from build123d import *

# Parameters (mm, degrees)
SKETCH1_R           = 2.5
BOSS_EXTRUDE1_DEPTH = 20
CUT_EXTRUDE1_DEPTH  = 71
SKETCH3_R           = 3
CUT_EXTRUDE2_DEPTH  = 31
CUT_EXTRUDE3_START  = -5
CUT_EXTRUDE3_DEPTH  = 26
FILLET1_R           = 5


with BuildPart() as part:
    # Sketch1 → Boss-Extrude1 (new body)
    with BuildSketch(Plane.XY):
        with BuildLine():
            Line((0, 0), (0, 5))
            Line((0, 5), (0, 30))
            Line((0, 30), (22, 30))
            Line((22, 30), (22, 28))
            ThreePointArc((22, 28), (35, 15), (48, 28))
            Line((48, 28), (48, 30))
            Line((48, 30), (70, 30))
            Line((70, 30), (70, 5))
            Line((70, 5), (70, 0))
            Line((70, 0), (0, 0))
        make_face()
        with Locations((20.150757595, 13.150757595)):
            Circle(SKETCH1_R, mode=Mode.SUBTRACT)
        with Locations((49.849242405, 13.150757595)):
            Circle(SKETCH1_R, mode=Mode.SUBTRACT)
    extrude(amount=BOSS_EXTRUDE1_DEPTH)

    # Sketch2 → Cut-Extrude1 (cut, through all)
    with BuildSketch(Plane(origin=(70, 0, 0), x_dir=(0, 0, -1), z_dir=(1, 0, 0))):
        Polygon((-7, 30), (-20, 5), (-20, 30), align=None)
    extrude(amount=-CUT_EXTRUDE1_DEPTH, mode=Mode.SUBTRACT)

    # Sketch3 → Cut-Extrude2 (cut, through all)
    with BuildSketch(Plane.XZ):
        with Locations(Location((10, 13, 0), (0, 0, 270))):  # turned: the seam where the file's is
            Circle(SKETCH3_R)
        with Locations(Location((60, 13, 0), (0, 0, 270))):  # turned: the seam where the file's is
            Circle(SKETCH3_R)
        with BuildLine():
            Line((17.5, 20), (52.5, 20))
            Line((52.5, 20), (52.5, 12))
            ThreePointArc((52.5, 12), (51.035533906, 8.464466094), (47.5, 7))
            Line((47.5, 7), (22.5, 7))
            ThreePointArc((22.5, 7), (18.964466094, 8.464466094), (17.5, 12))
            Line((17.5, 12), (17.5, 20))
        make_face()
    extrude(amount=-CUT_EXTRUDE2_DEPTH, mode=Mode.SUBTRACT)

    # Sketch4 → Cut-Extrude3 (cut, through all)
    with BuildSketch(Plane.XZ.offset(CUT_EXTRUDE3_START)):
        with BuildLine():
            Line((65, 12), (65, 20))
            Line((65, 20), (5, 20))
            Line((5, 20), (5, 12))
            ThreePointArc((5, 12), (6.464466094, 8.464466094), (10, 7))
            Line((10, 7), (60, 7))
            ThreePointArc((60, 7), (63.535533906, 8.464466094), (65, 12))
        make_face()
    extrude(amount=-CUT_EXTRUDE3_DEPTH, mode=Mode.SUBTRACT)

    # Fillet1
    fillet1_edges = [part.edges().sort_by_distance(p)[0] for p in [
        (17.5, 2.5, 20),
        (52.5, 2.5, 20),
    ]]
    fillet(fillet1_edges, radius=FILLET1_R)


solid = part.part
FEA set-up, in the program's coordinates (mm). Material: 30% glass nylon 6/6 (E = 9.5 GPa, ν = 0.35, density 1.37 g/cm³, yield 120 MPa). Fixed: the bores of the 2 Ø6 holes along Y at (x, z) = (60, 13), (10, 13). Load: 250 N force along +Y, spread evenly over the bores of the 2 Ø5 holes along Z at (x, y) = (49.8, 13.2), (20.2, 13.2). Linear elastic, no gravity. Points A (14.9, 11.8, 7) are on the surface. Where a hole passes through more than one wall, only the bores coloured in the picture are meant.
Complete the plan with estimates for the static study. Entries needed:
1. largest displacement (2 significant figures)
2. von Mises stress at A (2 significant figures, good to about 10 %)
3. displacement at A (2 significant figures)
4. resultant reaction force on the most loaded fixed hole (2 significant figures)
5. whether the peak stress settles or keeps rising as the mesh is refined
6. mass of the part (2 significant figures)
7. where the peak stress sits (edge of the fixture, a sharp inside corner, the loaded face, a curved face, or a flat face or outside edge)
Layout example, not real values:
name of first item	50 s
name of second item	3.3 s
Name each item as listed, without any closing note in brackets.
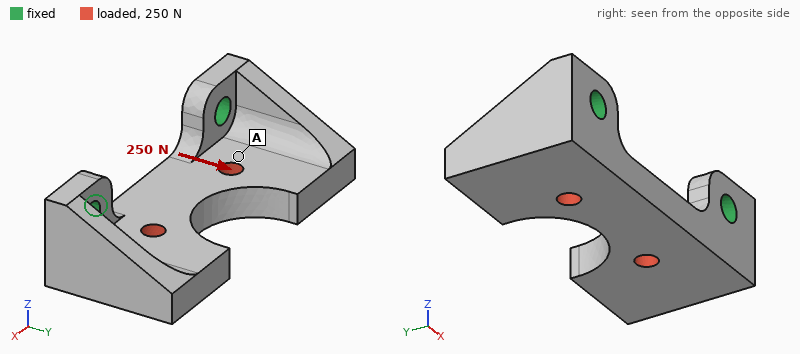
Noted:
largest displacement	46 µm
von Mises stress at A	1.7 MPa
displacement at A	17 µm
resultant reaction force on the most loaded fixed hole	130 N
whether the peak stress settles or keeps rising as the mesh is refined	keeps rising
mass of the part	22 g
where the peak stress sits	edge of the fixture
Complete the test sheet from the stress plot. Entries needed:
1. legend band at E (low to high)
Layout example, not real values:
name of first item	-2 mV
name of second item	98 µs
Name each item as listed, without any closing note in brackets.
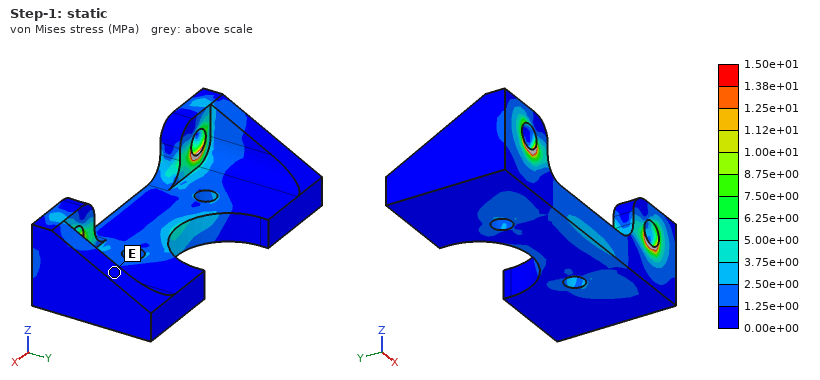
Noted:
legend band at E	0.00e+00 to 1.25e+00 MPa
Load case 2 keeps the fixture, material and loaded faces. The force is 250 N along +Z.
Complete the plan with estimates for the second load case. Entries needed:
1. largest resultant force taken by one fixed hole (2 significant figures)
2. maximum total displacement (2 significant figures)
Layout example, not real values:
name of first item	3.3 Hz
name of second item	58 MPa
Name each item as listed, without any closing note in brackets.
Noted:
largest resultant force taken by one fixed hole	150 N
maximum total displacement	95 µm
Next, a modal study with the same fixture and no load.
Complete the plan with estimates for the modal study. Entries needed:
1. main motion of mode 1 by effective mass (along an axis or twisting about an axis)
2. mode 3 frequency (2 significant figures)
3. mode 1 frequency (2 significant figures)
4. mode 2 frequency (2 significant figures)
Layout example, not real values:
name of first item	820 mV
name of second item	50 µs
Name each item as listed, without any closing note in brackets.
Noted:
main motion of mode 1 by effective mass	along Z
mode 3 frequency	5100 Hz
mode 1 frequency	2500 Hz
mode 2 frequency	3200 Hz
